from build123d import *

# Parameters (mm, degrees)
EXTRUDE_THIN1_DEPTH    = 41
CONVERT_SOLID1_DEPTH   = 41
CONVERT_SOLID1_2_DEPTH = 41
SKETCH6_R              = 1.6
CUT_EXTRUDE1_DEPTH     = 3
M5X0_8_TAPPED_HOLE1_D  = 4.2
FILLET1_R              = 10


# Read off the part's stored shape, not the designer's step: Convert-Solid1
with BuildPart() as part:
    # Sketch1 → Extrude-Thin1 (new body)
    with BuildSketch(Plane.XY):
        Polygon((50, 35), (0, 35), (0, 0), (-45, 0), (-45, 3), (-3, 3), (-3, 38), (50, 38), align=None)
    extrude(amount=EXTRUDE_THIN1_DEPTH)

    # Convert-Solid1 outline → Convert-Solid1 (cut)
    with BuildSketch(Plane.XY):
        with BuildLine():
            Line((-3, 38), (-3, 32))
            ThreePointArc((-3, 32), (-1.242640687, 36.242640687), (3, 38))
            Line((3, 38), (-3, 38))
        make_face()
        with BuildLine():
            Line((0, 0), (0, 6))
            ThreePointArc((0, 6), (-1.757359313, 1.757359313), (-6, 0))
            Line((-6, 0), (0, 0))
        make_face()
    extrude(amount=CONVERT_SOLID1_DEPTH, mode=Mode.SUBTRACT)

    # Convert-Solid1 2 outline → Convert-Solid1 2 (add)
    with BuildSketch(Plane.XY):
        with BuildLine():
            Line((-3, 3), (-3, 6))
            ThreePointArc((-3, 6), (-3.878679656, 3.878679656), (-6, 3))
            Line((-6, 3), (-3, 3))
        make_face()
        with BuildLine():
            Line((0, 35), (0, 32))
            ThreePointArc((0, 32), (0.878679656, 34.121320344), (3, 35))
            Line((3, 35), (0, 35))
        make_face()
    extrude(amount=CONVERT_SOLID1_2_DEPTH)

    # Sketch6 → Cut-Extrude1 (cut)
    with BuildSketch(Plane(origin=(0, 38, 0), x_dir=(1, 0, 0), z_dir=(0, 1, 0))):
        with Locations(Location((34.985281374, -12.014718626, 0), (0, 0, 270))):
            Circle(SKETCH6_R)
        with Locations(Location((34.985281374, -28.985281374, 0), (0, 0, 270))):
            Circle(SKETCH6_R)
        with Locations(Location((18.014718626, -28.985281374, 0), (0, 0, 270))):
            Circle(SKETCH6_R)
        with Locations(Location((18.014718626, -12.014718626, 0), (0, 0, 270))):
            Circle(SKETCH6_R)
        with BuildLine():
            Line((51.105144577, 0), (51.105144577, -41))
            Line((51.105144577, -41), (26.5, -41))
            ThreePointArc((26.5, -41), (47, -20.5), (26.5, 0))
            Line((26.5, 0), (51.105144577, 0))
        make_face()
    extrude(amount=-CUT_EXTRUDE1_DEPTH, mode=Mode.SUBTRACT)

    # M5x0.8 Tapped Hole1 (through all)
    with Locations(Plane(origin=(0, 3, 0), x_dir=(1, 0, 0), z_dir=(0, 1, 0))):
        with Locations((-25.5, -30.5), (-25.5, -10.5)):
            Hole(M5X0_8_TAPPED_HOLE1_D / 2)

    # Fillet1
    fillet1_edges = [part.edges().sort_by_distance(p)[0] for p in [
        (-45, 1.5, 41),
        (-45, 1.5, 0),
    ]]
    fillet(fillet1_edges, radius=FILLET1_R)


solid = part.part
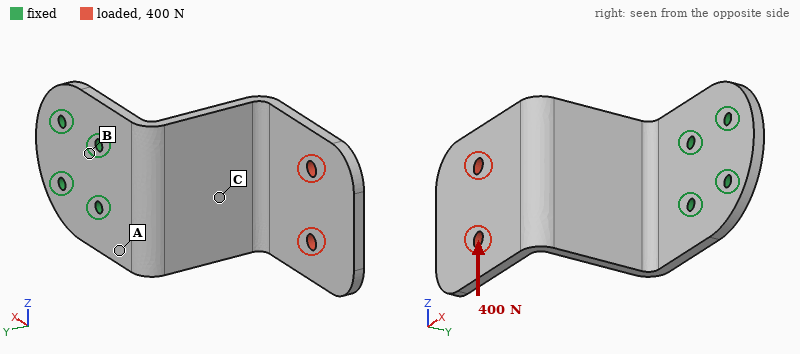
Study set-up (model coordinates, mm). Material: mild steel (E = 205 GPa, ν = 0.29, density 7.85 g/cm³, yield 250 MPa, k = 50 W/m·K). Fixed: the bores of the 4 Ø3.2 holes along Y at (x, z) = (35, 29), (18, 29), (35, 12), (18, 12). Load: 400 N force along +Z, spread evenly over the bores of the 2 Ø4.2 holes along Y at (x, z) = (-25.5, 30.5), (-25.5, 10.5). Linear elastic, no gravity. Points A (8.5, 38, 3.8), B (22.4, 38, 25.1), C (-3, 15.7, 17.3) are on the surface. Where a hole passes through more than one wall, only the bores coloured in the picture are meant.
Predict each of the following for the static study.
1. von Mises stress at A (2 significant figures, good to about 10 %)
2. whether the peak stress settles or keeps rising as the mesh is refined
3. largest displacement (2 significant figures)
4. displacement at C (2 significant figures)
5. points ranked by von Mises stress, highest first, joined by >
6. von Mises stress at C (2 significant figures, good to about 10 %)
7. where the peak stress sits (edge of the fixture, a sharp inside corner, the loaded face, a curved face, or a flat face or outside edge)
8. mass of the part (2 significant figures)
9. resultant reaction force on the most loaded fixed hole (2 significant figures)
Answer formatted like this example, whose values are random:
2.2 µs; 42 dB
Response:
46 MPa; keeps rising; 0.40 mm; 0.072 mm; C > A > B; 110 MPa; edge of the fixture; 110 g; 910 N
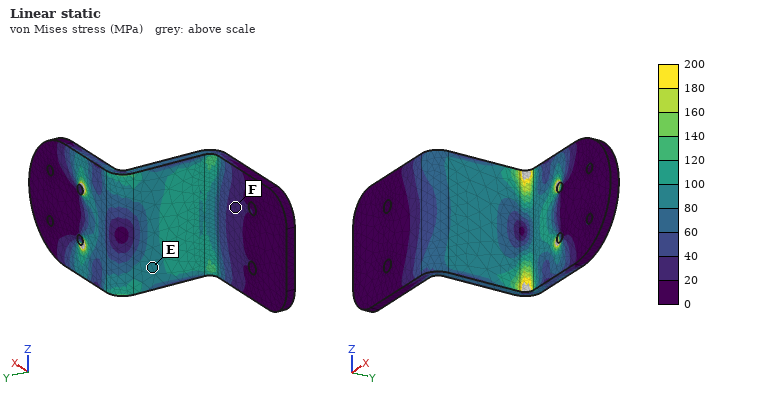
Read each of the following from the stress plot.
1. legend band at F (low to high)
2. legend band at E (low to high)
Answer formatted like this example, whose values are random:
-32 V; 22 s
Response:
20 to 40 MPa; 80 to 100 MPa
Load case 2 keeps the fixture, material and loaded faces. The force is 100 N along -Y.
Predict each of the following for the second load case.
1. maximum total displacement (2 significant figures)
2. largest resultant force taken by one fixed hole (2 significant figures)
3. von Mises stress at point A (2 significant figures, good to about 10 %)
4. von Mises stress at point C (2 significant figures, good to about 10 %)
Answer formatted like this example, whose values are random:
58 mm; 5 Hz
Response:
0.45 mm; 91 N; 51 MPa; 36 MPa
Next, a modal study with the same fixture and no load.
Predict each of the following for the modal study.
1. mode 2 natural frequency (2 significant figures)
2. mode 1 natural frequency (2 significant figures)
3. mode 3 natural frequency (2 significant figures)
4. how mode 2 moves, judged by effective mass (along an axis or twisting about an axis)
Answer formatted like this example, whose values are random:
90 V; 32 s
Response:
920 Hz; 380 Hz; 1400 Hz; along Z
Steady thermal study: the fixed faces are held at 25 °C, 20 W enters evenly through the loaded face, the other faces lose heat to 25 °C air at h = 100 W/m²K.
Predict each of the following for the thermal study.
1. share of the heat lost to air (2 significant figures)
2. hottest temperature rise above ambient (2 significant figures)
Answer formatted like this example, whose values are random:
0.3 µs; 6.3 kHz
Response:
93 %; 60 K
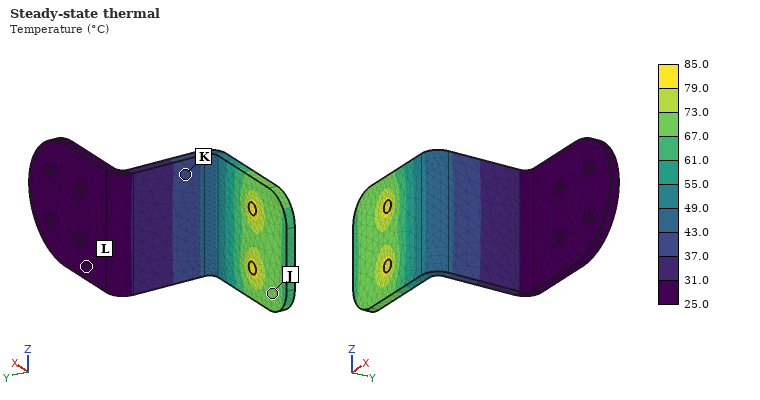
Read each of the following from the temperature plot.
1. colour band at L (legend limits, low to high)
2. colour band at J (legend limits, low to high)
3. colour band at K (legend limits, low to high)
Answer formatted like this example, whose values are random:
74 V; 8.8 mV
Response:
25.0 to 31.0 °C; 67.0 to 73.0 °C; 37.0 to 43.0 °C
